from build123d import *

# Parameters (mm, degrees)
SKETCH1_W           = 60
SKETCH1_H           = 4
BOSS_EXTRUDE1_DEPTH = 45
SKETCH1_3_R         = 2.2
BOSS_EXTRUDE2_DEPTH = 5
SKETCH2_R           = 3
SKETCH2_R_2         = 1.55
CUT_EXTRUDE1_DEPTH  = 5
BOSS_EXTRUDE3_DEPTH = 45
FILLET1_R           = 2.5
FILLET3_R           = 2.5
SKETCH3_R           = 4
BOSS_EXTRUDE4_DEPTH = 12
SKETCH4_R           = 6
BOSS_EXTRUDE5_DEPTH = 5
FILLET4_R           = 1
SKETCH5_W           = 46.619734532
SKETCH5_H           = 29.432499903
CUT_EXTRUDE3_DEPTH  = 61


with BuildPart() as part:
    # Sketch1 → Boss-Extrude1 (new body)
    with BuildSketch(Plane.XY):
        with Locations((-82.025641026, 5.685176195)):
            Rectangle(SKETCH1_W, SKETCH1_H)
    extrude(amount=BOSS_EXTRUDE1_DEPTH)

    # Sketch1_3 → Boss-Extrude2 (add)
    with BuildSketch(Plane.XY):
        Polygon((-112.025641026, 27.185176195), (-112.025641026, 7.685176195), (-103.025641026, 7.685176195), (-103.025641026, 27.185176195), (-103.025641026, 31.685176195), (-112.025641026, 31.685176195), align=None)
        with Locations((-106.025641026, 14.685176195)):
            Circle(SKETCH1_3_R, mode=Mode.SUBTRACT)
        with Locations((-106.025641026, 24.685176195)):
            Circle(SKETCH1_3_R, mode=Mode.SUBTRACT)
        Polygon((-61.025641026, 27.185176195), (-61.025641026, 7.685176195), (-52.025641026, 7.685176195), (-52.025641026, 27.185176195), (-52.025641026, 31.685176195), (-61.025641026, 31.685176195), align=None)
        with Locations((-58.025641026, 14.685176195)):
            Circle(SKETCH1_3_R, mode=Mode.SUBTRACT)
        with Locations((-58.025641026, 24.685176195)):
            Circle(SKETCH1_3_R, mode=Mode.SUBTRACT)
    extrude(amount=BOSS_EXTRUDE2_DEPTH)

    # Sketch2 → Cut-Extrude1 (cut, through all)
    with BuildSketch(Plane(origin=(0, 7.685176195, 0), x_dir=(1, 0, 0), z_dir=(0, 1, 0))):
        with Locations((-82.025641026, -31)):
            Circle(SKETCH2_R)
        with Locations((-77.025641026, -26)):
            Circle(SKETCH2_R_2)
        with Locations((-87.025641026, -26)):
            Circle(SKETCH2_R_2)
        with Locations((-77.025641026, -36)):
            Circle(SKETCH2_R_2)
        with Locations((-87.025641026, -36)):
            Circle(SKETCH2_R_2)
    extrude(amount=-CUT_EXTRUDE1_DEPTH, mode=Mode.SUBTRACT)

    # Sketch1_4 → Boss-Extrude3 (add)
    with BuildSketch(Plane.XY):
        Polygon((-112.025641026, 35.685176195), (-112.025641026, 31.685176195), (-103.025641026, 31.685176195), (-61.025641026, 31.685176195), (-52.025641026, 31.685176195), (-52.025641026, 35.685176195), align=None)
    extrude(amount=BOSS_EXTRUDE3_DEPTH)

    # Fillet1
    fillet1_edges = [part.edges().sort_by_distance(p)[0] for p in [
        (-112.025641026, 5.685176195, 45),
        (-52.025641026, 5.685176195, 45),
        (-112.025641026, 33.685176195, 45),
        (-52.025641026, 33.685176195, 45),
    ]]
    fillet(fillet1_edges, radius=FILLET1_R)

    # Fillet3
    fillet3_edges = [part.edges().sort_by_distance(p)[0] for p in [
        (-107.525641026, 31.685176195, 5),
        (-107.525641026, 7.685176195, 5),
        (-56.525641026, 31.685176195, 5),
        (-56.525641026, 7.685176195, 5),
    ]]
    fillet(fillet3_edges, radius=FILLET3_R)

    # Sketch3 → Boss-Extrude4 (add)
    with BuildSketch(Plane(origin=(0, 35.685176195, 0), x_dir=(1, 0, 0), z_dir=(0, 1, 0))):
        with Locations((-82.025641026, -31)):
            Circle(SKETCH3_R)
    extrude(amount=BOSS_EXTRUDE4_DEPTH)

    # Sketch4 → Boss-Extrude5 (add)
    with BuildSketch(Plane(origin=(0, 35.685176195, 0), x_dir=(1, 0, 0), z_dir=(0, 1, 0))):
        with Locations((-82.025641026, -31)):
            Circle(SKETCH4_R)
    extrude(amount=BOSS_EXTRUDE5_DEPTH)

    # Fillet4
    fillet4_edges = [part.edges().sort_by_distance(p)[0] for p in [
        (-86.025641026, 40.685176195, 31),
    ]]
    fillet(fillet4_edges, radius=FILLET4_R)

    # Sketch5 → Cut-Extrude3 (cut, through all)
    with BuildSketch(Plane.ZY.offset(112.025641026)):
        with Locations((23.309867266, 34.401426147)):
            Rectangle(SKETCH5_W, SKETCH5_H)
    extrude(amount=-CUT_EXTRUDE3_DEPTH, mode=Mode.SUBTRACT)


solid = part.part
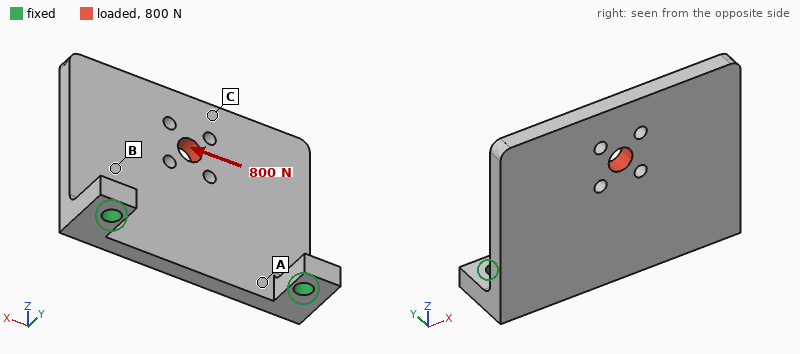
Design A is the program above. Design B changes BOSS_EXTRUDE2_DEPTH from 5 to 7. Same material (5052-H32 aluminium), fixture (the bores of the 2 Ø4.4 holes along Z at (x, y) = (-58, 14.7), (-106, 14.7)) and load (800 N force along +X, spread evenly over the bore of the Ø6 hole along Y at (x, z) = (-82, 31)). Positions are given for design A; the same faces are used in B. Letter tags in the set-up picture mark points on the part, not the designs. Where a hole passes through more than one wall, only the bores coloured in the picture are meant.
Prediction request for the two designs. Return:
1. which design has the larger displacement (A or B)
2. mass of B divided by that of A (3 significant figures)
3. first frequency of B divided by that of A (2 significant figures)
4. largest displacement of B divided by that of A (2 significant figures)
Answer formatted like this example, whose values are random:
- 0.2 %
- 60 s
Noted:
- A
- 1.03
- 1.3
- 0.59
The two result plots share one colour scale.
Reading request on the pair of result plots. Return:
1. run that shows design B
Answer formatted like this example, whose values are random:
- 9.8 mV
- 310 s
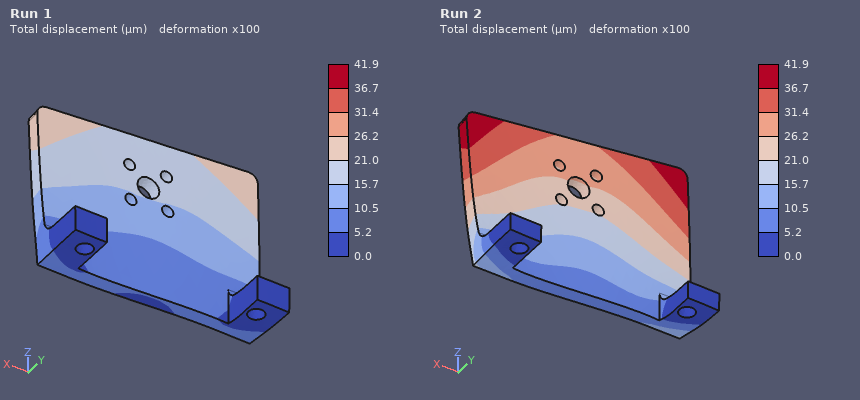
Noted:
- Run 1
